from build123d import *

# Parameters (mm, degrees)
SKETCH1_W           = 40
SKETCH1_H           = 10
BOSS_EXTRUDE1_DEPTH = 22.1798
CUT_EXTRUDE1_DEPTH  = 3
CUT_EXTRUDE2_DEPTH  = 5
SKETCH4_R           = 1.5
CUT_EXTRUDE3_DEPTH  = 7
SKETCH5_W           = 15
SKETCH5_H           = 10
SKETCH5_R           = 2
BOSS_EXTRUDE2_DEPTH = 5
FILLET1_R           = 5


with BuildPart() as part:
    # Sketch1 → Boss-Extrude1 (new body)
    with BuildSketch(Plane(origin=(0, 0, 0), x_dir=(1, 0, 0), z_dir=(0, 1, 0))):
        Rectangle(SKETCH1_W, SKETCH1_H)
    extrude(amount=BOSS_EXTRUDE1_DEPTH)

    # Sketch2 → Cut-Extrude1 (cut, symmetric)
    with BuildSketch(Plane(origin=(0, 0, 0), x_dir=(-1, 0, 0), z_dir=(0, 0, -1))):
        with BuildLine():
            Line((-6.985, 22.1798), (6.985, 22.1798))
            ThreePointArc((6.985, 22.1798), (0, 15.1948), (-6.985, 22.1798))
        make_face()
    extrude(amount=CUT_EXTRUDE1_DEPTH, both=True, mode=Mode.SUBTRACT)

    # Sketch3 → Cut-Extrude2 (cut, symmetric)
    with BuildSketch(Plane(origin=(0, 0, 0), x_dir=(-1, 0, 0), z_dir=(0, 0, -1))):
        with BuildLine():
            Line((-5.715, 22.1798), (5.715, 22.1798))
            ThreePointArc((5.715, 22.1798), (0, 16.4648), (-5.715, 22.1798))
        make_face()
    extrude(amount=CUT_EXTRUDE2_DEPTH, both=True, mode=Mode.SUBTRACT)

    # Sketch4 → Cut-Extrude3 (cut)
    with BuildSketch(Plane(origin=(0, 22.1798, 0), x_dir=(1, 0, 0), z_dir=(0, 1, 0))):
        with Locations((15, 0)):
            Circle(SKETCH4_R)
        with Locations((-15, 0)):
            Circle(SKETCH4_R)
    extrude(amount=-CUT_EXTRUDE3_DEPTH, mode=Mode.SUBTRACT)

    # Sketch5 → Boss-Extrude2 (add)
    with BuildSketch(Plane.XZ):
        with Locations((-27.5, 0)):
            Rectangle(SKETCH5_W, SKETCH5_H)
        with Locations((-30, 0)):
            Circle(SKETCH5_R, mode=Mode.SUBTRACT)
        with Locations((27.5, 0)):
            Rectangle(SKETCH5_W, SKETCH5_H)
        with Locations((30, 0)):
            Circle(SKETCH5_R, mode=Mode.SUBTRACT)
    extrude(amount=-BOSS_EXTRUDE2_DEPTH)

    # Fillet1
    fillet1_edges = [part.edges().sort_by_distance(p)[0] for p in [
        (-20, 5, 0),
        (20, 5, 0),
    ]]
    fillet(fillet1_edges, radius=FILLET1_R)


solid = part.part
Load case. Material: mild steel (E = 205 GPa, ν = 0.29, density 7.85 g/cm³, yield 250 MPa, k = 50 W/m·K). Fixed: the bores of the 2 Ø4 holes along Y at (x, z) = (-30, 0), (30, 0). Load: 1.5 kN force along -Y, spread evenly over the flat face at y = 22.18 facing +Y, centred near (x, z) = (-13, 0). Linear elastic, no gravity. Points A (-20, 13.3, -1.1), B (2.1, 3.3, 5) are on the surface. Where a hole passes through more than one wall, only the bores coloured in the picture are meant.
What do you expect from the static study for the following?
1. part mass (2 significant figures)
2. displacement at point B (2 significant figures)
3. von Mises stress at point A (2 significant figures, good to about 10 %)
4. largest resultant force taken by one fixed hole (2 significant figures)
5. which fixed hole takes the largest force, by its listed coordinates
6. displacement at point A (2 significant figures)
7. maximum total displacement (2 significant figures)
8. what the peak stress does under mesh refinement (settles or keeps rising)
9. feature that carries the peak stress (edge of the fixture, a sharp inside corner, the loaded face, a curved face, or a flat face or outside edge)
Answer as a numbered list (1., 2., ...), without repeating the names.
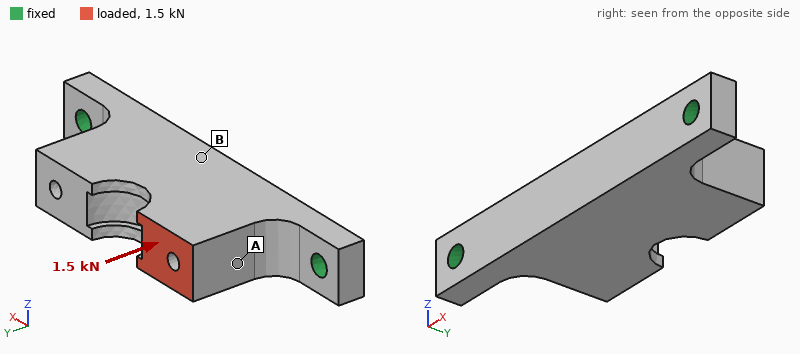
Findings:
1. 75 g
2. 6.0 µm
3. 19 MPa
4. 1.3 kN
5. (-30, 0)
6. 7.7 µm
7. 8.3 µm
8. keeps rising
9. edge of the fixture
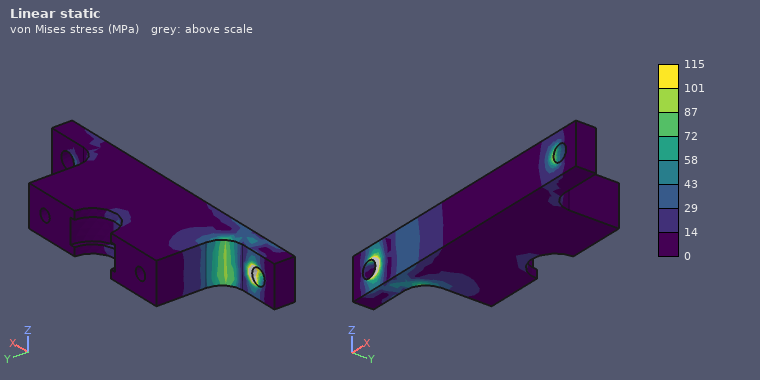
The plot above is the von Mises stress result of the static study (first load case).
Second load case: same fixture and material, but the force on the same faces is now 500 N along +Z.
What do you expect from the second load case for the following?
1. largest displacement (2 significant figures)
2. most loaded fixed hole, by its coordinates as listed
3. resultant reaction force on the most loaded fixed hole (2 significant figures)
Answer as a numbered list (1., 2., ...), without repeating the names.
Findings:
1. 42 µm
2. (-30, 0)
3. 380 N
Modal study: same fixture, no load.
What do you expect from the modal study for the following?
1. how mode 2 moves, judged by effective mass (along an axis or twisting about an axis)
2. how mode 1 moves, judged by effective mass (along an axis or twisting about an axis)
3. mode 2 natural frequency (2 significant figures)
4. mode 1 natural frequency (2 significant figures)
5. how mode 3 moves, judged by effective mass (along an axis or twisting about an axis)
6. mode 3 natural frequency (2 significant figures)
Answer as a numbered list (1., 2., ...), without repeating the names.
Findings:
1. along Y
2. along Z
3. 9700 Hz
4. 4200 Hz
5. along Z
6. 12 kHz
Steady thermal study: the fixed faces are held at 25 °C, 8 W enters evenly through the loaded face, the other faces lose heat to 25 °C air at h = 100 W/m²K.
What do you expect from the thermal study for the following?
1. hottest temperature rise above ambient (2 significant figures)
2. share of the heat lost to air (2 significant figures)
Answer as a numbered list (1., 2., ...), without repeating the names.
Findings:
1. 27 K
2. 47 %
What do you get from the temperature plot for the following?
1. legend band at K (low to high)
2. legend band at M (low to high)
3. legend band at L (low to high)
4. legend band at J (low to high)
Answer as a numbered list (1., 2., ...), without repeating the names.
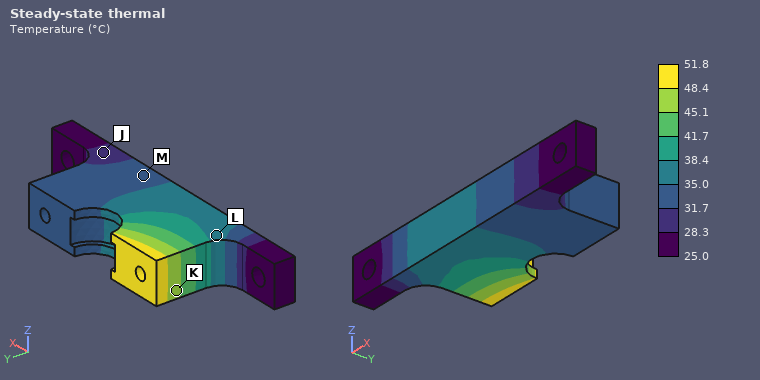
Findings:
1. 45.1 to 48.4 °C
2. 31.7 to 35.0 °C
3. 35.0 to 38.4 °C
4. 28.3 to 31.7 °C
